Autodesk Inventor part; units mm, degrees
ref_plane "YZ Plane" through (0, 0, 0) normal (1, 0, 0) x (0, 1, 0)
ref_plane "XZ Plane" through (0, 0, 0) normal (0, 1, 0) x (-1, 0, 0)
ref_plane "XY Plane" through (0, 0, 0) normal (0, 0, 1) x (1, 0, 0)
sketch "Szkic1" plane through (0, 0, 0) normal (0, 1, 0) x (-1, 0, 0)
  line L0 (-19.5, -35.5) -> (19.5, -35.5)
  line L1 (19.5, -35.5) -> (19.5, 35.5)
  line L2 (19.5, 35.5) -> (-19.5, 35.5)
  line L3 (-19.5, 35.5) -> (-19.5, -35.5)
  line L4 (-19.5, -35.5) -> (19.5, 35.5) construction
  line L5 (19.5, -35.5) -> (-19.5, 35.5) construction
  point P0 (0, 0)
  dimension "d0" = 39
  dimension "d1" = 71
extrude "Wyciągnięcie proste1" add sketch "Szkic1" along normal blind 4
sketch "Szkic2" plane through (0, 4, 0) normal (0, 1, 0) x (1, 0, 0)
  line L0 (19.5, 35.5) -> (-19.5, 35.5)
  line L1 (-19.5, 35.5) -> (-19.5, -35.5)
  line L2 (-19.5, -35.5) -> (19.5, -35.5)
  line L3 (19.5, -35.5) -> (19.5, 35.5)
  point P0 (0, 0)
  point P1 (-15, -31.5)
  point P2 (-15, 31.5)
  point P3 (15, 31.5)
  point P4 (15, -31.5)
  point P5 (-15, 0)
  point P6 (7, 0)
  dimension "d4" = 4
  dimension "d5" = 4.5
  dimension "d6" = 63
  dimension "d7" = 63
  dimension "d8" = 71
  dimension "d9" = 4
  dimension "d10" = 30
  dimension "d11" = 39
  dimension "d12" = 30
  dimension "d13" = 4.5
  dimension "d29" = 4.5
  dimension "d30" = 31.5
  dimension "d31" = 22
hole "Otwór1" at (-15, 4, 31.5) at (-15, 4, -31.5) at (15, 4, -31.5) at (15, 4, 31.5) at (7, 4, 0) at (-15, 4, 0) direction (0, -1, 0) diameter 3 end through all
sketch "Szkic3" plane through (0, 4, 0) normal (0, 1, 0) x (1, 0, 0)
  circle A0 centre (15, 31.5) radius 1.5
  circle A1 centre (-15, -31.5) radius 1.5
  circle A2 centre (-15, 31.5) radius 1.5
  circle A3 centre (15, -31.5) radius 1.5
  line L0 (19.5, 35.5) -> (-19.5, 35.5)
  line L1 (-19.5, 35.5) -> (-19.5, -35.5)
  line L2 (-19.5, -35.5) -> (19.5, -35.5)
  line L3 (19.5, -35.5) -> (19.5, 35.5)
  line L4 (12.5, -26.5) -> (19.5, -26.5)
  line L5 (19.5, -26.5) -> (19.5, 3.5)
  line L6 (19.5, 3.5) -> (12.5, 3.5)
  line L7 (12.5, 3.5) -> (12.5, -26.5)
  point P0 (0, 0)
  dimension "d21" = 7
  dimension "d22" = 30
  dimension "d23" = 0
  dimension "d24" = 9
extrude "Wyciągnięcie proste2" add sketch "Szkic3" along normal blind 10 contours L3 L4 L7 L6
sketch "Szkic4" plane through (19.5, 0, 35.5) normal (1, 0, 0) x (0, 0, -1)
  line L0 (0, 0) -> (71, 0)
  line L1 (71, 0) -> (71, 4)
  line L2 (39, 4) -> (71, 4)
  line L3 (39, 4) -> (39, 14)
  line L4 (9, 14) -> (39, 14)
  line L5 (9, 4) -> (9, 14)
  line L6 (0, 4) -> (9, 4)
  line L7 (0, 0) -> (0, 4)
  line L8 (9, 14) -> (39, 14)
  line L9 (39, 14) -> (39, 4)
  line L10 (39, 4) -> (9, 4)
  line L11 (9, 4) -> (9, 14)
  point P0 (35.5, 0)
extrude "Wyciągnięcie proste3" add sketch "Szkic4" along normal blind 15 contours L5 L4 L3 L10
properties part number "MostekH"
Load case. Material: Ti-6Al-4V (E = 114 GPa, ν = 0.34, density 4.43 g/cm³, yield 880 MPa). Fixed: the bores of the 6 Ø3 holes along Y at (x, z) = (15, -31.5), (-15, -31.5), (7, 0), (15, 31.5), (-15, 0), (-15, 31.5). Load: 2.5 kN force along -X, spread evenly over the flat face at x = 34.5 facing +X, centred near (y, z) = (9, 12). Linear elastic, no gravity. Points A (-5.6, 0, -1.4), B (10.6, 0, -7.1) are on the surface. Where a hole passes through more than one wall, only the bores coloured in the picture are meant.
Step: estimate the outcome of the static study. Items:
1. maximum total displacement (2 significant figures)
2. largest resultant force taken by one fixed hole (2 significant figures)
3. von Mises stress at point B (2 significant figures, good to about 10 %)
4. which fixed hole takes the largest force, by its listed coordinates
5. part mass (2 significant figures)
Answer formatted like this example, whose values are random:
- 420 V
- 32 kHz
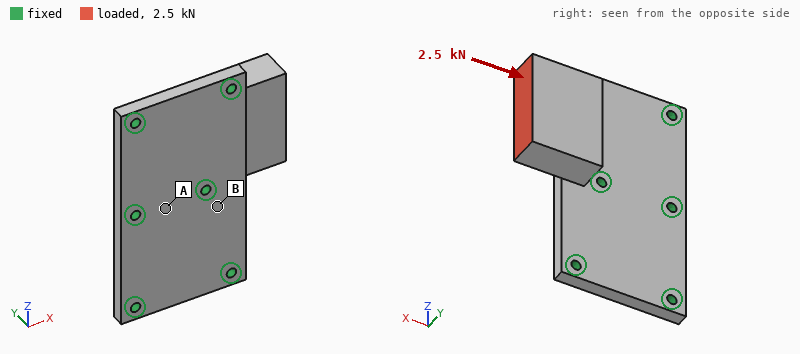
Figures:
- 0.12 mm
- 1.2 kN
- 60 MPa
- (7, 0)
- 78 g
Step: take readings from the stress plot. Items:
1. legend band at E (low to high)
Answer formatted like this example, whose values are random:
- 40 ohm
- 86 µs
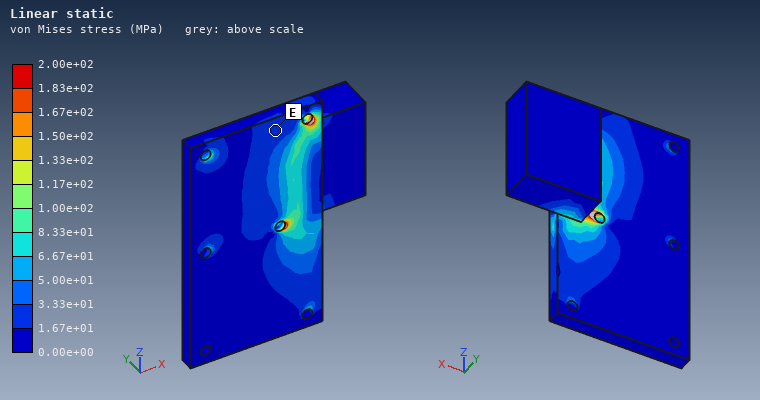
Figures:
- 1.67e+01 to 3.33e+01 MPa
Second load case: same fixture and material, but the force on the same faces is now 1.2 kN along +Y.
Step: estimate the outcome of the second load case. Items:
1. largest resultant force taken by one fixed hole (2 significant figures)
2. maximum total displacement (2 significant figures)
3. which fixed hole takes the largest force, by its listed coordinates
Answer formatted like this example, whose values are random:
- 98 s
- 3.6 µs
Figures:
- 1.1 kN
- 0.20 mm
- (15, 31.5)
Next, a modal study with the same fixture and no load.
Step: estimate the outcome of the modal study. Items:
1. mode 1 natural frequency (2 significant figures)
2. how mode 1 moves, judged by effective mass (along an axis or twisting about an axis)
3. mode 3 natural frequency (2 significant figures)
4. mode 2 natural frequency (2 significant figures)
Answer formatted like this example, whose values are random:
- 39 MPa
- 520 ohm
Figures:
- 3800 Hz
- along Y
- 15 kHz
- 14 kHz
